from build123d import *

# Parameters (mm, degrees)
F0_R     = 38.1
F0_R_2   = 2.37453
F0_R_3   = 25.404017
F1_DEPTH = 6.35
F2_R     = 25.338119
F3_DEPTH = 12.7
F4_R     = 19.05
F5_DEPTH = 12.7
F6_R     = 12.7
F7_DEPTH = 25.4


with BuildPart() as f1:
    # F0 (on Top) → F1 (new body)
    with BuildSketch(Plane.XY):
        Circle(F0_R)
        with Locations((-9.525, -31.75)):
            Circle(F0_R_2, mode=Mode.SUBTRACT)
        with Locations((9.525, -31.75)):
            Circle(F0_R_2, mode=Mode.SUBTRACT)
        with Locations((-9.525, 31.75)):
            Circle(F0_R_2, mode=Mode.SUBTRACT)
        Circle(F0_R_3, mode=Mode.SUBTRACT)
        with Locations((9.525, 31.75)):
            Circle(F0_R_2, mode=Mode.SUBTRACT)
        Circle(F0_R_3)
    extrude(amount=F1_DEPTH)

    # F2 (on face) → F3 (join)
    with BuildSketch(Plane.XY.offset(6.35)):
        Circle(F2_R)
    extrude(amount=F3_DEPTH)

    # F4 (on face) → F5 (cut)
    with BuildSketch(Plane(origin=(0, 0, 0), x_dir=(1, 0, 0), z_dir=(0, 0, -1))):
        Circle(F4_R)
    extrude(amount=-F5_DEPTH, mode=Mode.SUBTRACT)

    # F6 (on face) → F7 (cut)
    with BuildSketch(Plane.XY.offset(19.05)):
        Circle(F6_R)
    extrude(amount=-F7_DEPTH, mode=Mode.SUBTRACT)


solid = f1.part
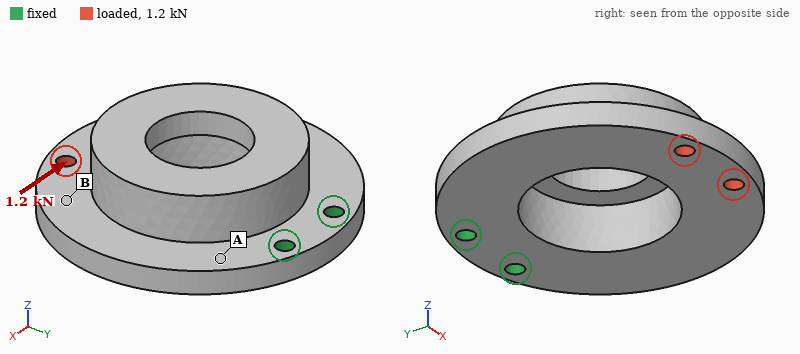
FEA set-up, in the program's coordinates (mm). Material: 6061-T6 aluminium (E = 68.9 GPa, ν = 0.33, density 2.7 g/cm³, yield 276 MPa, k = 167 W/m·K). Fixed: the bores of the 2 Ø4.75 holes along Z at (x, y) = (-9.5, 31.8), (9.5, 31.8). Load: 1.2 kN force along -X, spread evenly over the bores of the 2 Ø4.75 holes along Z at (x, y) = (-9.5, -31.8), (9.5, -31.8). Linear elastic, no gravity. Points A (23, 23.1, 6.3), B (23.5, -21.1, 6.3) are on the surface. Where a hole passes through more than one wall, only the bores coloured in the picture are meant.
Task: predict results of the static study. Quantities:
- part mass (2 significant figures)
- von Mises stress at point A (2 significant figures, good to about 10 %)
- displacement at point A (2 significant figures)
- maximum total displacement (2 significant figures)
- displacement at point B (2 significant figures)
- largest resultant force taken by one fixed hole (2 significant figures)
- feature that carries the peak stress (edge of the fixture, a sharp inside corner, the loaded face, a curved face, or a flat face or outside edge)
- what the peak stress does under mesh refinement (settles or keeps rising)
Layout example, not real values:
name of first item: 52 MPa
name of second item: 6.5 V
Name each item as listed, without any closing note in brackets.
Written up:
part mass: 98 g
von Mises stress at point A: 28 MPa
displacement at point A: 0.028 mm
maximum total displacement: 0.13 mm
displacement at point B: 0.10 mm
largest resultant force taken by one fixed hole: 3.2 kN
feature that carries the peak stress: edge of the fixture
what the peak stress does under mesh refinement: keeps rising
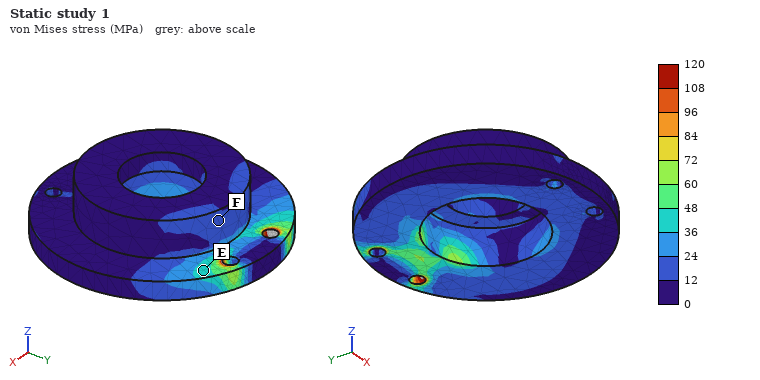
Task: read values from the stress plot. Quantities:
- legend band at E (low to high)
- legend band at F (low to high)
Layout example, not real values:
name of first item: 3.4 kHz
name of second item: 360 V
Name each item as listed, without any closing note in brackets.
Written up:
legend band at E: 36 to 48 MPa
legend band at F: 12 to 24 MPa
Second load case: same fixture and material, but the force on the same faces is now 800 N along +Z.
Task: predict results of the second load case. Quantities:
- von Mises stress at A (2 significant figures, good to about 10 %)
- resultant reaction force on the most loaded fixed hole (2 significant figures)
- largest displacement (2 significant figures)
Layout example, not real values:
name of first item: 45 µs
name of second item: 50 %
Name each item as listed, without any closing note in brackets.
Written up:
von Mises stress at A: 54 MPa
resultant reaction force on the most loaded fixed hole: 930 N
largest displacement: 0.70 mm
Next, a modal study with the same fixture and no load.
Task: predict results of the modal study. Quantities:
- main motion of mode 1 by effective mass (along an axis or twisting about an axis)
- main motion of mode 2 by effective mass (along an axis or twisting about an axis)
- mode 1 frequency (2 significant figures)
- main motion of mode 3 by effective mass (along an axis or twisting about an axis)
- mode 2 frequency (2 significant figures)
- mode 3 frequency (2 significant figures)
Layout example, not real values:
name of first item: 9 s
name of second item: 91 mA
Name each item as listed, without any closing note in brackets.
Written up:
main motion of mode 1 by effective mass: along Z
main motion of mode 2 by effective mass: along X
mode 1 frequency: 1100 Hz
main motion of mode 3 by effective mass: along X
mode 2 frequency: 2600 Hz
mode 3 frequency: 3400 Hz
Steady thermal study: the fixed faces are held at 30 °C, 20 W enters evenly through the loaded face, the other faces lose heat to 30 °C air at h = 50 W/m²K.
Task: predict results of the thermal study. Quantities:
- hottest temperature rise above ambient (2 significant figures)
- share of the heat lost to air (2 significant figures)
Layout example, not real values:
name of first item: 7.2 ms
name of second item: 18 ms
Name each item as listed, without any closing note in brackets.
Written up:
hottest temperature rise above ambient: 20 K
share of the heat lost to air: 29 %
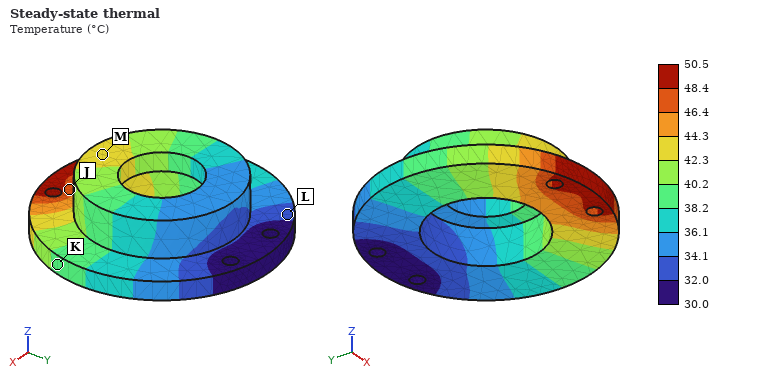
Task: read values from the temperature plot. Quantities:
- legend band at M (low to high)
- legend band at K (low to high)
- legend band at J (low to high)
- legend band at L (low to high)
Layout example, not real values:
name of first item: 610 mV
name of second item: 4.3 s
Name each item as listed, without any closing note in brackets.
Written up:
legend band at M: 42.3 to 44.3 °C
legend band at K: 38.2 to 40.2 °C
legend band at J: 46.4 to 48.4 °C
legend band at L: 32.0 to 34.1 °C
